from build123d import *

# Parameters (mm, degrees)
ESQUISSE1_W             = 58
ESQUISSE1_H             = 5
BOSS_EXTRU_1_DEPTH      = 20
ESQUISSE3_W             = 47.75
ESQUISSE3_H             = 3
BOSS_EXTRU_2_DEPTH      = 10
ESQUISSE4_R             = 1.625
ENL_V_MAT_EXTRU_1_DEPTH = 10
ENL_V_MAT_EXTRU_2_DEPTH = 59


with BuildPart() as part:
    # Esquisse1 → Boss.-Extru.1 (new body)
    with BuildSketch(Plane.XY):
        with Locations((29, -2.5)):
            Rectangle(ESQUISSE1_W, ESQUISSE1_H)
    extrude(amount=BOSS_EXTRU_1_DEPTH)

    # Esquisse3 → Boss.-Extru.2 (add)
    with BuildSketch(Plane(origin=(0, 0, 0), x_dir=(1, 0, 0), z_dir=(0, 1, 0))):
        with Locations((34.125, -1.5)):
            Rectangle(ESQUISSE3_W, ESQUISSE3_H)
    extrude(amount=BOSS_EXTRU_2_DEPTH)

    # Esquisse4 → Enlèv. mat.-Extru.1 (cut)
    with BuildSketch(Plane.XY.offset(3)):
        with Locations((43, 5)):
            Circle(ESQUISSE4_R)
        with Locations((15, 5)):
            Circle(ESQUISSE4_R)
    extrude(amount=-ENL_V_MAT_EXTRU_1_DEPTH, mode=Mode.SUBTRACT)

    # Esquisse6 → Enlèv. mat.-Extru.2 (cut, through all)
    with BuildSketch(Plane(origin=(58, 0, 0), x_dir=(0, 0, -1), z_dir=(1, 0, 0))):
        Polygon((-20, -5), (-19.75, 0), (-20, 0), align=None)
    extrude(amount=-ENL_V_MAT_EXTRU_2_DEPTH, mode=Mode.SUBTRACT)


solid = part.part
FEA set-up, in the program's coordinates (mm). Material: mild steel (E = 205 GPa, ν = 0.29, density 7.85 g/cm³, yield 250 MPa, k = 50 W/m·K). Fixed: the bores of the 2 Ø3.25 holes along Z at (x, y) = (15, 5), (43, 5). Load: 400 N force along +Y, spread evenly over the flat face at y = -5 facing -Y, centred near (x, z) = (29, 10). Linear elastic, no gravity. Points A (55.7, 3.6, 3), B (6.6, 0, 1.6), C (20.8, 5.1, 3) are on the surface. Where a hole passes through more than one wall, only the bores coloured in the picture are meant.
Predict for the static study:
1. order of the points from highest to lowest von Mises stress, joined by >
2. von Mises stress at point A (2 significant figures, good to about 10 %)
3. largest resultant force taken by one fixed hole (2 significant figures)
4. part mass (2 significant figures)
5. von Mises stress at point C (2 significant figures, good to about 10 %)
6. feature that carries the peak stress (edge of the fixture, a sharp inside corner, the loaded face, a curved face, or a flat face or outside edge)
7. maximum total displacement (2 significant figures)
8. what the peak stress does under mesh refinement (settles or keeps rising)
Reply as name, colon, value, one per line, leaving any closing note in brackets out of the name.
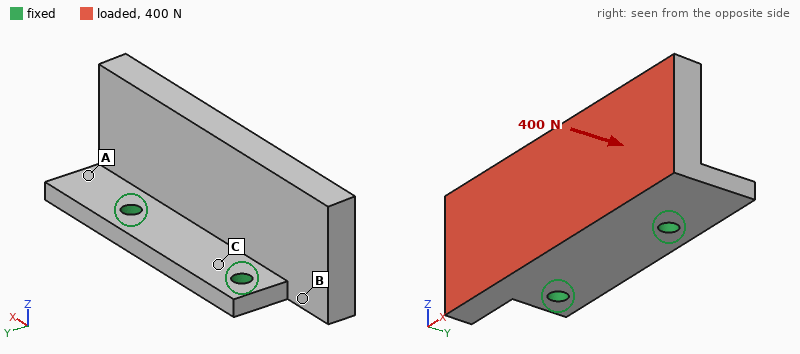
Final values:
order of the points from highest to lowest von Mises stress, joined by >: C > A > B
von Mises stress at point A: 21 MPa
largest resultant force taken by one fixed hole: 200 N
part mass: 56 g
von Mises stress at point C: 29 MPa
feature that carries the peak stress: edge of the fixture
maximum total displacement: 30 µm
what the peak stress does under mesh refinement: keeps rising
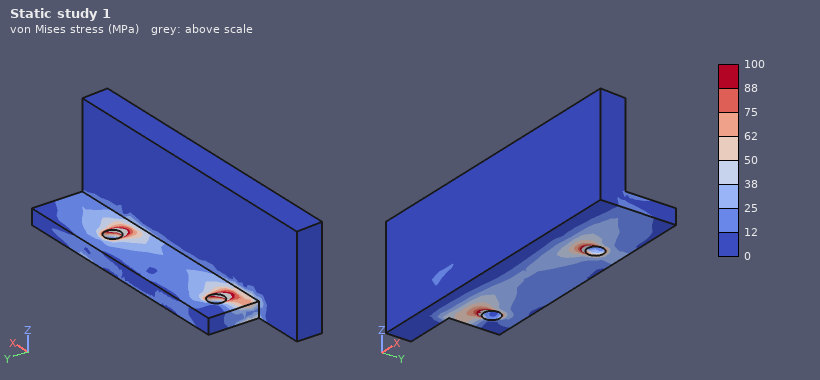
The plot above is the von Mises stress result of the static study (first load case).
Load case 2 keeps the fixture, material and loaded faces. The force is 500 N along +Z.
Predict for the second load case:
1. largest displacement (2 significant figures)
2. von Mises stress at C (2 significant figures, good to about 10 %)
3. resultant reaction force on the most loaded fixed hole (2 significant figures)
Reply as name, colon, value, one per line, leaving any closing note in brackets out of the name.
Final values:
largest displacement: 29 µm
von Mises stress at C: 32 MPa
resultant reaction force on the most loaded fixed hole: 250 N
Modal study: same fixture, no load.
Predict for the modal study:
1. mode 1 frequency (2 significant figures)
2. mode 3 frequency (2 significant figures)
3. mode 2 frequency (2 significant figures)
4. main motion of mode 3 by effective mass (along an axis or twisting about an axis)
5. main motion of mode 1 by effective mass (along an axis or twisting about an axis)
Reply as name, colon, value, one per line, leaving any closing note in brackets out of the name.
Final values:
mode 1 frequency: 3300 Hz
mode 3 frequency: 10 kHz
mode 2 frequency: 6200 Hz
main motion of mode 3 by effective mass: along X
main motion of mode 1 by effective mass: along Y
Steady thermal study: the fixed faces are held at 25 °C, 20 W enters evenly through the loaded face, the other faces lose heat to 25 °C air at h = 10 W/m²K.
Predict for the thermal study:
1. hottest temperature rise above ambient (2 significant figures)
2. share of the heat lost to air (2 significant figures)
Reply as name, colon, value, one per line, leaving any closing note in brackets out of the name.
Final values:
hottest temperature rise above ambient: 44 K
share of the heat lost to air: 4.0 %
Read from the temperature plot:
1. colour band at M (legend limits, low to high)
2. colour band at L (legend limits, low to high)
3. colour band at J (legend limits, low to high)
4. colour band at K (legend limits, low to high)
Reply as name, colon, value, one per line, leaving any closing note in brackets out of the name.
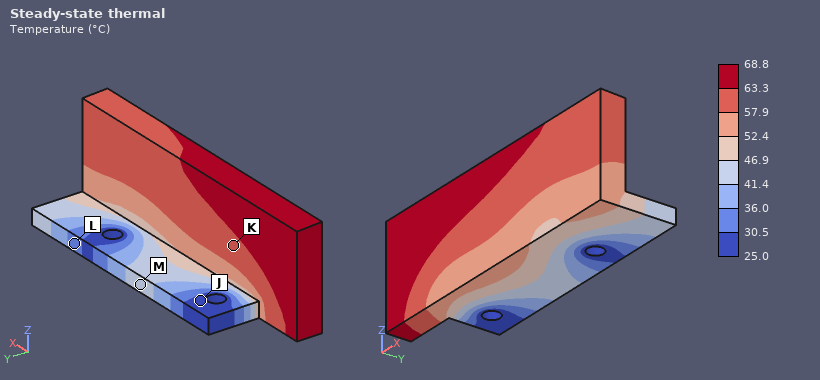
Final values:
colour band at M: 41.4 to 46.9 °C
colour band at L: 30.5 to 36.0 °C
colour band at J: 25.0 to 30.5 °C
colour band at K: 57.9 to 63.3 °C
